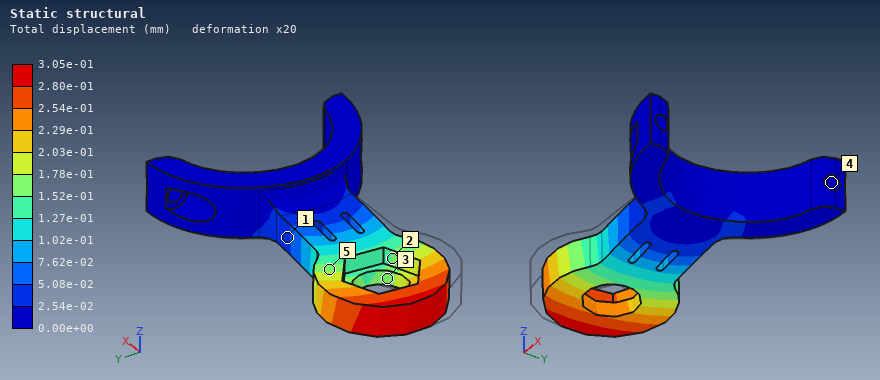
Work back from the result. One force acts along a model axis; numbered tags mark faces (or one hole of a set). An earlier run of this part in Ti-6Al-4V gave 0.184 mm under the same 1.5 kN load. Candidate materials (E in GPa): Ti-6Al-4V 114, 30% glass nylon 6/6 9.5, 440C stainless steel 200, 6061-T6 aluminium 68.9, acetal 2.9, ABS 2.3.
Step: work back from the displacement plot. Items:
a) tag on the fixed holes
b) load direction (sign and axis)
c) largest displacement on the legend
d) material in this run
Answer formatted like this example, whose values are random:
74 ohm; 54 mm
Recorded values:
4; +Y; 3.05e-01 mm; 6061-T6 aluminium
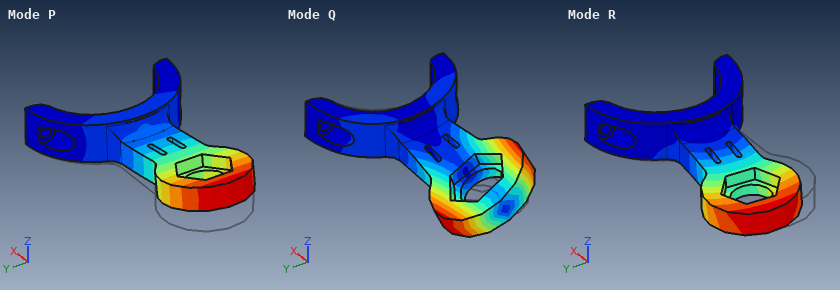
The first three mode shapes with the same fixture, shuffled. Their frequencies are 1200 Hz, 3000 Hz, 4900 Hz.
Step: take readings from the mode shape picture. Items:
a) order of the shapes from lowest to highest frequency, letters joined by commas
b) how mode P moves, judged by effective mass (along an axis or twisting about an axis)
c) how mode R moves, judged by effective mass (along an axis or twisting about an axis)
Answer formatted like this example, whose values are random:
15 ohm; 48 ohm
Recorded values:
P, R, Q; along Z; along Y
